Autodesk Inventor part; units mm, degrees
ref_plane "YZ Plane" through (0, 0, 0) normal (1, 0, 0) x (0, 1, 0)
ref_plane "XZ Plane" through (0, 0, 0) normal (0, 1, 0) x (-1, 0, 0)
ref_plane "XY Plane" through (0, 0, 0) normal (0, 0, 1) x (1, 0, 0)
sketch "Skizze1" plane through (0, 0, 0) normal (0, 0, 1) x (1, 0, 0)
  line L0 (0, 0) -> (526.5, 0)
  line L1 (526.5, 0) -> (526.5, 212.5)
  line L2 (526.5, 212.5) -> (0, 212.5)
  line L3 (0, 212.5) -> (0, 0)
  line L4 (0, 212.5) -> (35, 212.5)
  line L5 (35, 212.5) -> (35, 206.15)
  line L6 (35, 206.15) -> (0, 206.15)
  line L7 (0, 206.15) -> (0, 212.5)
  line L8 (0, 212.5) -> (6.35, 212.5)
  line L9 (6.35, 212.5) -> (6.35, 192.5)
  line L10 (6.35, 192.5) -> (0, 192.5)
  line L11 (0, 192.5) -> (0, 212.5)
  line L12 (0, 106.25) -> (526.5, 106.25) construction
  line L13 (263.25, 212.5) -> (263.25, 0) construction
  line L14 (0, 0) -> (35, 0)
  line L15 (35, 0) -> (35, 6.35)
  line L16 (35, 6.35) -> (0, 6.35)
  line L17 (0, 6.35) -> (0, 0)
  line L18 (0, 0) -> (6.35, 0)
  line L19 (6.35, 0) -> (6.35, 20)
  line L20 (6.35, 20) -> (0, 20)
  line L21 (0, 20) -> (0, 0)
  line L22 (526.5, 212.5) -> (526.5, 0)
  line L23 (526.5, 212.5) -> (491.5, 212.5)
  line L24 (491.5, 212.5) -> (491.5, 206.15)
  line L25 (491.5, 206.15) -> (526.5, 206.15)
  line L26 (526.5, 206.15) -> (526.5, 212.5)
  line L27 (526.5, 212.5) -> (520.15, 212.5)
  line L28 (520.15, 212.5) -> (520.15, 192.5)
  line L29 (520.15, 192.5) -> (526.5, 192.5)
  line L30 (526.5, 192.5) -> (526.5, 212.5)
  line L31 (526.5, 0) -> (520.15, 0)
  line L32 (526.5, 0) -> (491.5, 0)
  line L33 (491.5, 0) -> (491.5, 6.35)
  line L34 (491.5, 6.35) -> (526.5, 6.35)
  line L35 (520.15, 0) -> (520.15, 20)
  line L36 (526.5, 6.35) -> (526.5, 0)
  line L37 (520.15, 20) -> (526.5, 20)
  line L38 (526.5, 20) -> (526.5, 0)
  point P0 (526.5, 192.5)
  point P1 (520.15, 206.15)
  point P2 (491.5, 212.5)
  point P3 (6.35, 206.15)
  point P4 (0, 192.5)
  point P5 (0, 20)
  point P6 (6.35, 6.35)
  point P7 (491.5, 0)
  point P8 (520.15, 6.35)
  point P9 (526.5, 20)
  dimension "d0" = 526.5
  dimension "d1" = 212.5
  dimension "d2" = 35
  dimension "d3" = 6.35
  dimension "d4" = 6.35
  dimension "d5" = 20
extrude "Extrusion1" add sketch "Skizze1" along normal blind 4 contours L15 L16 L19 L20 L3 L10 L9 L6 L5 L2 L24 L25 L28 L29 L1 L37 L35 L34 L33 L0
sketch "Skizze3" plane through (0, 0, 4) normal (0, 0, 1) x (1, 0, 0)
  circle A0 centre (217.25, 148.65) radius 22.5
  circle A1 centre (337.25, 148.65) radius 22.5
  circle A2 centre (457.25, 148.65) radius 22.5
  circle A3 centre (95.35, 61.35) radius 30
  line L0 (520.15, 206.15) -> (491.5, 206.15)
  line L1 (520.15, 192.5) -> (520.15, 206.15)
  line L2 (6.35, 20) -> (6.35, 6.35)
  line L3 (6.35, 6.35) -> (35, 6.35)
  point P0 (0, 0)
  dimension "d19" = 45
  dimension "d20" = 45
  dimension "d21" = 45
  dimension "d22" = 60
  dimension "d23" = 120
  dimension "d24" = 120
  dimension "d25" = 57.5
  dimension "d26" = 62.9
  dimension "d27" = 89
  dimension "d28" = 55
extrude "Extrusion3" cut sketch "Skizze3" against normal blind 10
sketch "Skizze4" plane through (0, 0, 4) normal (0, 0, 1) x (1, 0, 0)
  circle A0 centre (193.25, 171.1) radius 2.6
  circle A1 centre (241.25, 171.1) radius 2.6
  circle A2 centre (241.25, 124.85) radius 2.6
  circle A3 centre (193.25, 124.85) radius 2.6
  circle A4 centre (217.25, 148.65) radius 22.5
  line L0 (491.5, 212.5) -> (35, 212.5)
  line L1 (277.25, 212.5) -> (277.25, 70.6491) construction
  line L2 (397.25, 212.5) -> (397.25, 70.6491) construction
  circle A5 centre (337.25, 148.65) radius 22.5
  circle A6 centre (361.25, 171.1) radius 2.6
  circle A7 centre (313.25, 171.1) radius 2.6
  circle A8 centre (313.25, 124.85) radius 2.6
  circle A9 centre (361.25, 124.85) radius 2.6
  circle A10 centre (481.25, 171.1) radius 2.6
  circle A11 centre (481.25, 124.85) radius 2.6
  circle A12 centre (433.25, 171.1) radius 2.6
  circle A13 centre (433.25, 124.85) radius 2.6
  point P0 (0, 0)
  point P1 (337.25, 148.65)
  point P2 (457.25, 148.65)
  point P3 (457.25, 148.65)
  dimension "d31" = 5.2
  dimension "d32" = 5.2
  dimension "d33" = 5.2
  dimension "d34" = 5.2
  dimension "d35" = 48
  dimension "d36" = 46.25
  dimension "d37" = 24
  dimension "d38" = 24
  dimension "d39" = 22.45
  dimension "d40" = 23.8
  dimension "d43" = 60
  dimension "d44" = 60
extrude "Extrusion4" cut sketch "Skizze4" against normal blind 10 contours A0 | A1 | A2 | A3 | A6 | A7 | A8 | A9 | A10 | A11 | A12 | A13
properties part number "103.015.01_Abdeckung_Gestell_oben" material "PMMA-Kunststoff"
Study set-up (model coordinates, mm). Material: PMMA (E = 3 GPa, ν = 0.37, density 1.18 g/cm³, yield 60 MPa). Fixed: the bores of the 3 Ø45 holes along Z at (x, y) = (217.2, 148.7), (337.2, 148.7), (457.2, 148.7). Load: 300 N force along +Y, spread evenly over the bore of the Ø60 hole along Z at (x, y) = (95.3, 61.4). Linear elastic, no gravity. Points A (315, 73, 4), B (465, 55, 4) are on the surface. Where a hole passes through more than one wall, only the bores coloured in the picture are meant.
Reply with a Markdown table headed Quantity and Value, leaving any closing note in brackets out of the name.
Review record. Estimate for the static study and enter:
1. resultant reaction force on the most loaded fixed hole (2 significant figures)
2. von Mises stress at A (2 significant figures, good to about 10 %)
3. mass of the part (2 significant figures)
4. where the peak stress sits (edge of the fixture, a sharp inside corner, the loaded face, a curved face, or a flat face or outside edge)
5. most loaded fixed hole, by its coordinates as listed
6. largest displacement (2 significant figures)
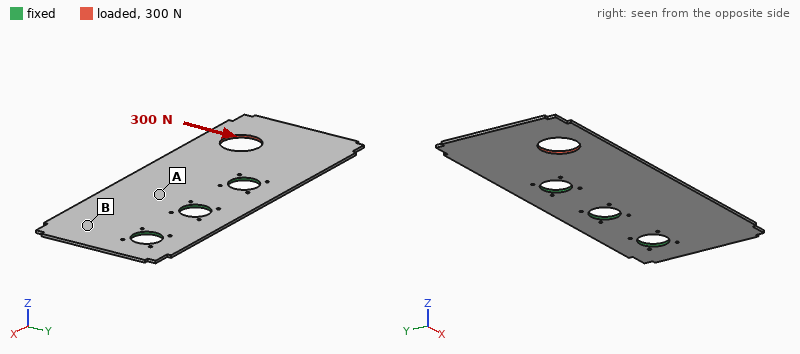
| Quantity | Value |
|---|---|
| resultant reaction force on the most loaded fixed hole | 430 N |
| von Mises stress at A | 0.40 MPa |
| mass of the part | 490 g |
| where the peak stress sits | a curved face |
| most loaded fixed hole, by its coordinates as listed | (217.2, 148.7) |
| largest displacement | 0.18 mm |
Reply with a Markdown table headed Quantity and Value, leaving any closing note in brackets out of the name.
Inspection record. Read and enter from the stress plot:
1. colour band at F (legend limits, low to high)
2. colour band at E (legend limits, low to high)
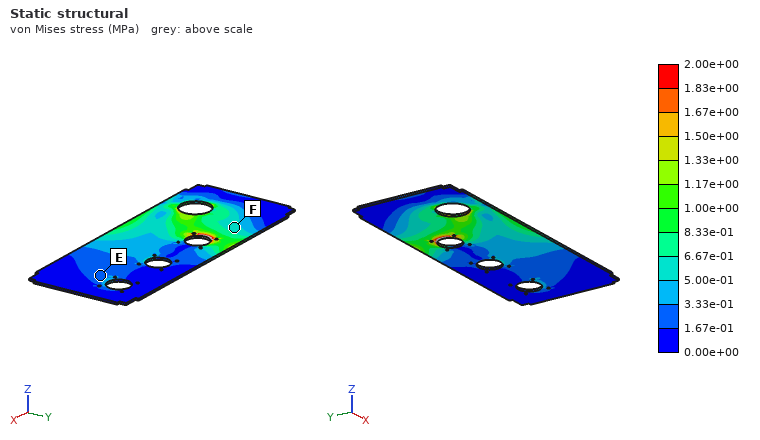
| Quantity | Value |
|---|---|
| colour band at F | 5.00e-01 to 6.67e-01 MPa |
| colour band at E | 1.67e-01 to 3.33e-01 MPa |
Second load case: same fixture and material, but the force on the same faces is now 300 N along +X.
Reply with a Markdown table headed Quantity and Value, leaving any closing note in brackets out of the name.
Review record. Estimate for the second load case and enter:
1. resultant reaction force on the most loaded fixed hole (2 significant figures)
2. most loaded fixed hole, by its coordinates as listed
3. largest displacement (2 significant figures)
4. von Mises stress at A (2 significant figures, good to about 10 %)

| Quantity | Value |
|---|---|
| resultant reaction force on the most loaded fixed hole | 190 N |
| most loaded fixed hole, by its coordinates as listed | (217.2, 148.7) |
| largest displacement | 0.10 mm |
| von Mises stress at A | 0.36 MPa |
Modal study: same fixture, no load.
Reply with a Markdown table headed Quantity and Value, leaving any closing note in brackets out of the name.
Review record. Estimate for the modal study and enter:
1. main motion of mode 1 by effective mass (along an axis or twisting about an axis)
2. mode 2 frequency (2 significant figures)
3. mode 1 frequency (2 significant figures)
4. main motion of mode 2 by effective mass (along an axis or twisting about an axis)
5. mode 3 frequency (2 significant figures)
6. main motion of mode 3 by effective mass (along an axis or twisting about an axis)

| Quantity | Value |
|---|---|
| main motion of mode 1 by effective mass | along Z |
| mode 2 frequency | 46 Hz |
| mode 1 frequency | 24 Hz |
| main motion of mode 2 by effective mass | twisting about X |
| mode 3 frequency | 66 Hz |
| main motion of mode 3 by effective mass | along Z |
